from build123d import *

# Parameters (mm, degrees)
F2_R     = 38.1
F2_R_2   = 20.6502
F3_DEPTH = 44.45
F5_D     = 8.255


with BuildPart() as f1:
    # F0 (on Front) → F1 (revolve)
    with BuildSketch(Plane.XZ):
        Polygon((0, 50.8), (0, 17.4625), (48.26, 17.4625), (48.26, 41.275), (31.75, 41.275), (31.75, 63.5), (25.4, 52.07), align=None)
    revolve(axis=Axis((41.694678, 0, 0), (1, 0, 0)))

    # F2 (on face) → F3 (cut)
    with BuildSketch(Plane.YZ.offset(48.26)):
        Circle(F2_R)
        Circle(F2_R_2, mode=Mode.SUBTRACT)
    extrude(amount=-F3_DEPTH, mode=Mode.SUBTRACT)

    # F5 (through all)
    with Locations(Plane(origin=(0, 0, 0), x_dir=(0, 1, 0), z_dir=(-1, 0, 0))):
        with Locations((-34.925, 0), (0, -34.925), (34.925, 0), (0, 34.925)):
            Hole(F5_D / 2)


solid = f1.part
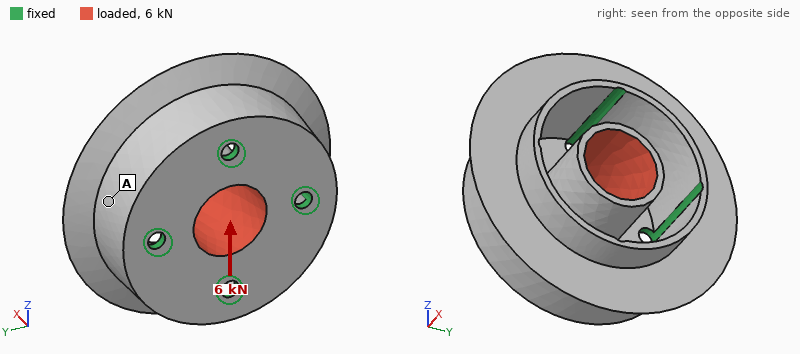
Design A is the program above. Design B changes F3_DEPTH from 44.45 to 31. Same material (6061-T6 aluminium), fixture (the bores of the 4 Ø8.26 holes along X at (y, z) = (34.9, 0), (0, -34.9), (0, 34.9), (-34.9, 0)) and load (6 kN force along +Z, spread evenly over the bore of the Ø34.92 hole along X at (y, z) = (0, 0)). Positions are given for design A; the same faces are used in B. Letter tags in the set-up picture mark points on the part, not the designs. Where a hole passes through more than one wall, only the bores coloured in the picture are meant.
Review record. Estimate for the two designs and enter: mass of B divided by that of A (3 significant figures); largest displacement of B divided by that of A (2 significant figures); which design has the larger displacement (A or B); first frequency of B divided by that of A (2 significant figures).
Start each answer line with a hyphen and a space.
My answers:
- 1.23
- 0.12
- A
- 2.3
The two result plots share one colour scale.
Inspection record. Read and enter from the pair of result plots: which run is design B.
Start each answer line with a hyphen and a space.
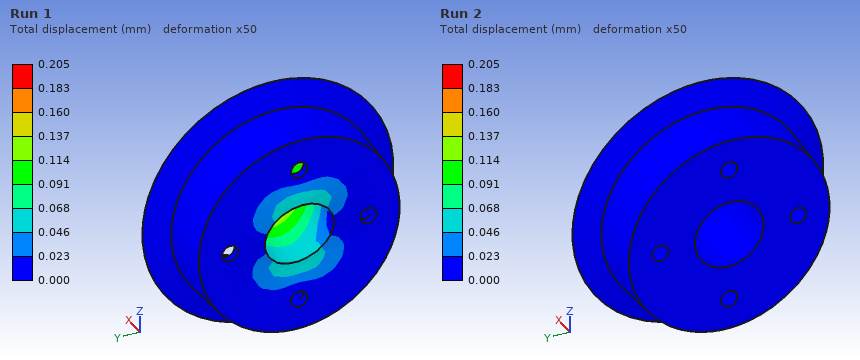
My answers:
- Run 2
